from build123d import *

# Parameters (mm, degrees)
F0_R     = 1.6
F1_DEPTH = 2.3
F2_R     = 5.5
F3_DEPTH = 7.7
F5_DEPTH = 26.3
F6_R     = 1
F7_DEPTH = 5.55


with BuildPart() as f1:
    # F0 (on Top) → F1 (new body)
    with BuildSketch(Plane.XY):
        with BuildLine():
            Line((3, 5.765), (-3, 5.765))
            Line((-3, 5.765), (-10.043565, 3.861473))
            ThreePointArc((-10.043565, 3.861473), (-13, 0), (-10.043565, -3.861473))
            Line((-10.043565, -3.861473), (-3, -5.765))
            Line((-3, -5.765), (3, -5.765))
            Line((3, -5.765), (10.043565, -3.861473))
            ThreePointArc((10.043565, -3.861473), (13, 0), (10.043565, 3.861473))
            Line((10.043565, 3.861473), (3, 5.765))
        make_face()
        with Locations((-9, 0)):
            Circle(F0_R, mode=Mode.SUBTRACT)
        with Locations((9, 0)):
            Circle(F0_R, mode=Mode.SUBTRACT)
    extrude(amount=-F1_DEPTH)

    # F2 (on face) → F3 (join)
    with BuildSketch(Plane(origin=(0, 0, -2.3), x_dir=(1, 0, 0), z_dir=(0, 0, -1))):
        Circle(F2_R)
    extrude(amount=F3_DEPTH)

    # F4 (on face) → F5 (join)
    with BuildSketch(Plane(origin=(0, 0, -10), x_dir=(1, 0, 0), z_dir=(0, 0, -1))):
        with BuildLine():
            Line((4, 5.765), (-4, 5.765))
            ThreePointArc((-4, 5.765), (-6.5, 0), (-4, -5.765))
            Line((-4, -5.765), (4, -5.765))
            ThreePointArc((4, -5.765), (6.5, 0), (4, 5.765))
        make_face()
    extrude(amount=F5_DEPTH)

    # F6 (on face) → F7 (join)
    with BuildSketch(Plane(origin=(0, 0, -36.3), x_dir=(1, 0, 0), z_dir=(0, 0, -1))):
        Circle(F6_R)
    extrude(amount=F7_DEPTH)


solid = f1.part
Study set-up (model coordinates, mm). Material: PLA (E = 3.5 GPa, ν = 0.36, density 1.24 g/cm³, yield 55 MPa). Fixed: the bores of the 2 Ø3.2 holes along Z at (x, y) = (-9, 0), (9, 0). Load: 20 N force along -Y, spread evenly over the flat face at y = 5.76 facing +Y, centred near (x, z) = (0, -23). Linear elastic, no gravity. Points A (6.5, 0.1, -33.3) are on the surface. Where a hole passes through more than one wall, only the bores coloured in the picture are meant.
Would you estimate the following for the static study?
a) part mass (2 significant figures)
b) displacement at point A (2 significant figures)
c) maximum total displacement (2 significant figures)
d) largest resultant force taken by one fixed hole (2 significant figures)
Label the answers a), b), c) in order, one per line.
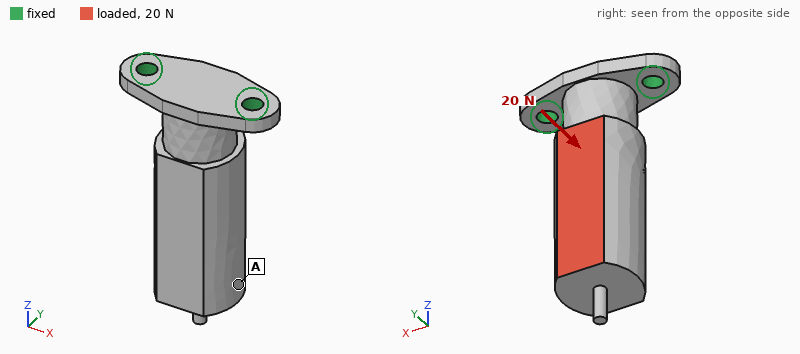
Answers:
a) 5.9 g
b) 0.48 mm
c) 0.61 mm
d) 10 N
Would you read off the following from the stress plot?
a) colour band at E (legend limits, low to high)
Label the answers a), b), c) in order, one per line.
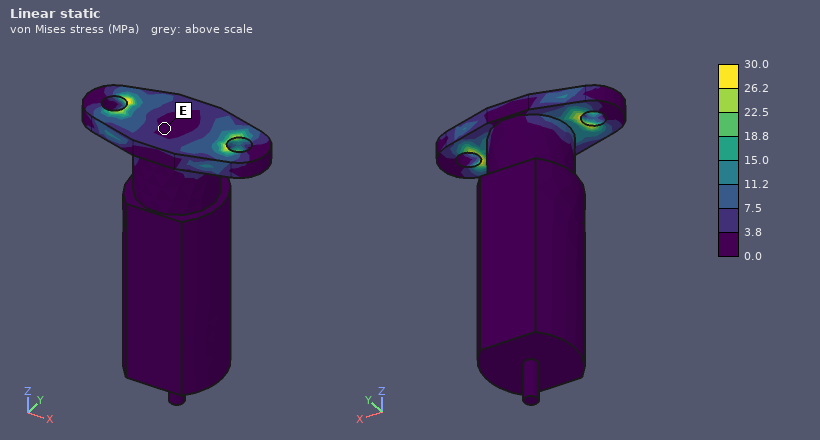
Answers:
a) 0.0 to 3.8 MPa
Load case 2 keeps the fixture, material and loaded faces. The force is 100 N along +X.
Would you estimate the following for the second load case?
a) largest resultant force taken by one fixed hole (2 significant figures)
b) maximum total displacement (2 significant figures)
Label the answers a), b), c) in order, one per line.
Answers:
a) 170 N
b) 0.59 mm
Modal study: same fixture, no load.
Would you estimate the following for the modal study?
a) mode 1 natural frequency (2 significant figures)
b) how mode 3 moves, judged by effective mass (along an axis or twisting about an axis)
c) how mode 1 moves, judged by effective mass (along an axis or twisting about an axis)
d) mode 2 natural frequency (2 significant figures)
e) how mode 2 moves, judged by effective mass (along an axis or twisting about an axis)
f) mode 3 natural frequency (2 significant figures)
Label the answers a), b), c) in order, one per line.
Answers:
a) 560 Hz
b) along Z
c) along Y
d) 1300 Hz
e) along X
f) 4700 Hz
